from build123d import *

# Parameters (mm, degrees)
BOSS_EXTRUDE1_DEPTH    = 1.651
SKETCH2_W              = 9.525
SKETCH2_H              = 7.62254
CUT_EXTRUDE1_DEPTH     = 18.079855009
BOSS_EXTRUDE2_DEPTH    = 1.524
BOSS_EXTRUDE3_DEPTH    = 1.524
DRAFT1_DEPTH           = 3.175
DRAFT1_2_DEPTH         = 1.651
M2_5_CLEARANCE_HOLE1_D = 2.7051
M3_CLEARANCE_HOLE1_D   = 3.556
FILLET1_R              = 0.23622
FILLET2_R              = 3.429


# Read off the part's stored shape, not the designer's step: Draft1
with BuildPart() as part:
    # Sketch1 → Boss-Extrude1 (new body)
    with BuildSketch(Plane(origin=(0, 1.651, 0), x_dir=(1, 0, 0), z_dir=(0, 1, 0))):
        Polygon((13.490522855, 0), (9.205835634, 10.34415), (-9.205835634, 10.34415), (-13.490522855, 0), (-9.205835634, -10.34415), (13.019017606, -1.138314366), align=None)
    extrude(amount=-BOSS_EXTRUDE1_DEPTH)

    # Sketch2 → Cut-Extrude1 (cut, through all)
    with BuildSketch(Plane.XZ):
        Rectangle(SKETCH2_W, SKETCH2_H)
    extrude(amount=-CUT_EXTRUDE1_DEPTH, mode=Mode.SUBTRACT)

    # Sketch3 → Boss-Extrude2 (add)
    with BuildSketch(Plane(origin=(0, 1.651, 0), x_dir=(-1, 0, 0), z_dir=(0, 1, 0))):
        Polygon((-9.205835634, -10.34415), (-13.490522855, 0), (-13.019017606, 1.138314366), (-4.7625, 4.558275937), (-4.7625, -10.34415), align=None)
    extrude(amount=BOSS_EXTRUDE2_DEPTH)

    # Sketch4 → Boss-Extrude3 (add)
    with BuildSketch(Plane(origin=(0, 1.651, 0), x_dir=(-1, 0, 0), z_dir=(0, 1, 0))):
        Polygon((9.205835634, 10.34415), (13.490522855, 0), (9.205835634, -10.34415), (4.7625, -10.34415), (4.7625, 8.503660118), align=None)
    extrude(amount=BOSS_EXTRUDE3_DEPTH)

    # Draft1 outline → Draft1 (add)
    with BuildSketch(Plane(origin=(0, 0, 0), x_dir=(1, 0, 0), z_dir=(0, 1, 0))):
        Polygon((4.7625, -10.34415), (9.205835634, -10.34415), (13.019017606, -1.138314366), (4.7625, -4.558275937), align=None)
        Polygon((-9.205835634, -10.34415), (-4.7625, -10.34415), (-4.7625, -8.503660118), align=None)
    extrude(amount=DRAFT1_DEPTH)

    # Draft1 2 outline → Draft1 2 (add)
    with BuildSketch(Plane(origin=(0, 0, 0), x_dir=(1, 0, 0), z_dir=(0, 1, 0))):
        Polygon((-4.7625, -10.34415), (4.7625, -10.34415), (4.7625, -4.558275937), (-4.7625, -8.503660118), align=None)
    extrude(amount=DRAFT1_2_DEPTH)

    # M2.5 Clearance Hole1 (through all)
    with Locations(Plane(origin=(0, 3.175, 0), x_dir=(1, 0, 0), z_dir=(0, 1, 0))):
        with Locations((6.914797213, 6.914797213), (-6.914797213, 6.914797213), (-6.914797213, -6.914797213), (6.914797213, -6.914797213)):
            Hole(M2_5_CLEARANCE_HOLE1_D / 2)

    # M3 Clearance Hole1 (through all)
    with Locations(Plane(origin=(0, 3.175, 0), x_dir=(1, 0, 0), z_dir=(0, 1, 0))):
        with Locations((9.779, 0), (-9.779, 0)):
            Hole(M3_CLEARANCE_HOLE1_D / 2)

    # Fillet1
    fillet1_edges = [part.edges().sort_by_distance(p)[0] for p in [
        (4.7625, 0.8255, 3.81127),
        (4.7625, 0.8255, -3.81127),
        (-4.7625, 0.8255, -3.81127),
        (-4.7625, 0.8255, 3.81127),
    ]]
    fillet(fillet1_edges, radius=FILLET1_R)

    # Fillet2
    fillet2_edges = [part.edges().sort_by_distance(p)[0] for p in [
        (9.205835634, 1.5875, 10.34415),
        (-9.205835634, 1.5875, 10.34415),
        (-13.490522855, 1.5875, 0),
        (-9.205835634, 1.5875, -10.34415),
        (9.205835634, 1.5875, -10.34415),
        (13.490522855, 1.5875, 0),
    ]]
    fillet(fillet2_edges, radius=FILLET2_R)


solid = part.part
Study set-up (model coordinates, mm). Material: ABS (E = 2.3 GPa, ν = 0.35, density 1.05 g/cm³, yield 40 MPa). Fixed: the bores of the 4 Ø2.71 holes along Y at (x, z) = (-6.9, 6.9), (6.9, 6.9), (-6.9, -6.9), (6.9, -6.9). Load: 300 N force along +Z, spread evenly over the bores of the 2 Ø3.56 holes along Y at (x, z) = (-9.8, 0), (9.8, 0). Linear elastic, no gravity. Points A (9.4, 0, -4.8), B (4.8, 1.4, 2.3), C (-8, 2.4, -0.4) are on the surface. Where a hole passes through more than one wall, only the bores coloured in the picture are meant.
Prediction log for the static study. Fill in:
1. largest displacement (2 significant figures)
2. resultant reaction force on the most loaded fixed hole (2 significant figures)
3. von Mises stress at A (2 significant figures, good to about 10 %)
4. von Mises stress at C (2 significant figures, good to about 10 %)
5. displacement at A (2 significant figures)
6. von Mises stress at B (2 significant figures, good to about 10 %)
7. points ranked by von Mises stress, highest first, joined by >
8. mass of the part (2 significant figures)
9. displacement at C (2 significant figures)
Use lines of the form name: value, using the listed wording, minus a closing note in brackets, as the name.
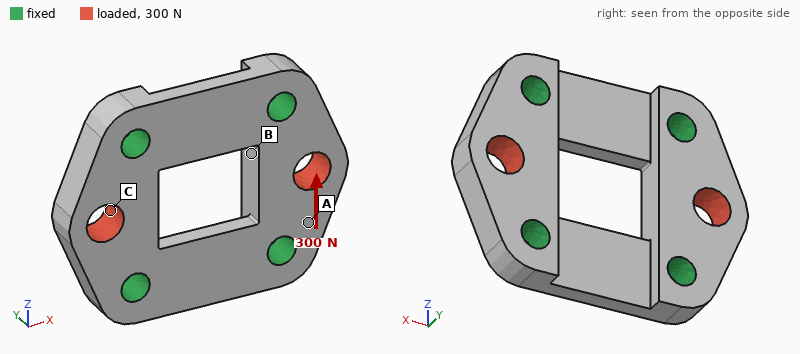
largest displacement: 23 µm
resultant reaction force on the most loaded fixed hole: 78 N
von Mises stress at A: 4.6 MPa
von Mises stress at C: 7.4 MPa
displacement at A: 7.5 µm
von Mises stress at B: 2.3 MPa
points ranked by von Mises stress, highest first, joined by >: C > A > B
mass of the part: 0.97 g
displacement at C: 9.2 µm
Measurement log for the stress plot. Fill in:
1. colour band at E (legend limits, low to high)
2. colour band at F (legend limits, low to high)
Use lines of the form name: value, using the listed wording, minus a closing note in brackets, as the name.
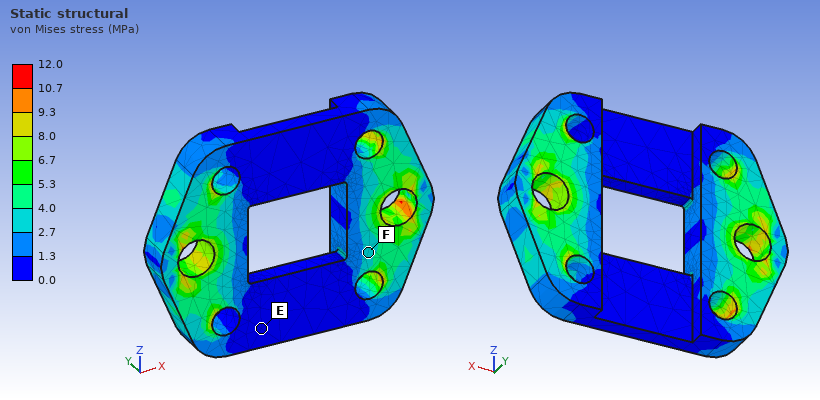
colour band at E: 0.0 to 1.3 MPa
colour band at F: 2.7 to 4.0 MPa
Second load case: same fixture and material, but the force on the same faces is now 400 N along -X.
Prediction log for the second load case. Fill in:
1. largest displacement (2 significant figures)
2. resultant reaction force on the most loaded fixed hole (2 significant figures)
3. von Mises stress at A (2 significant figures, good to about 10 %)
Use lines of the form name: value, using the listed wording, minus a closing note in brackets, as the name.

largest displacement: 44 µm
resultant reaction force on the most loaded fixed hole: 100 N
von Mises stress at A: 8.0 MPa
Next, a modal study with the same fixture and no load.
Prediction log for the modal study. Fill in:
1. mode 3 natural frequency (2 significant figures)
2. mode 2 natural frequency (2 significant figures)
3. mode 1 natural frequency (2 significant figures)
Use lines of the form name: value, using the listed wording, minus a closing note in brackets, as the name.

mode 3 natural frequency: 19 kHz
mode 2 natural frequency: 17 kHz
mode 1 natural frequency: 17 kHz
